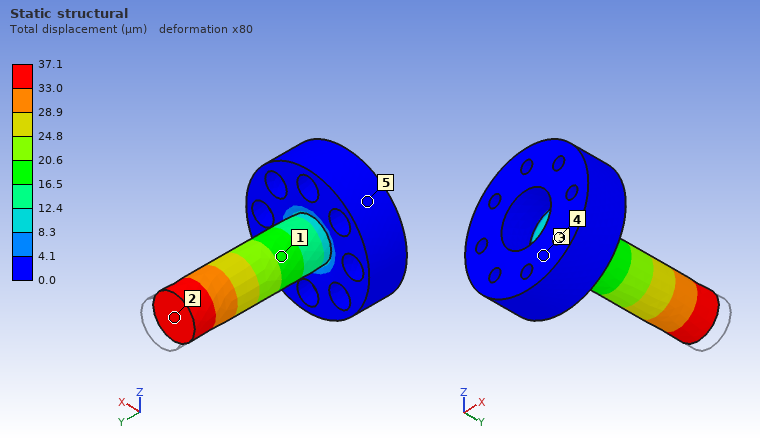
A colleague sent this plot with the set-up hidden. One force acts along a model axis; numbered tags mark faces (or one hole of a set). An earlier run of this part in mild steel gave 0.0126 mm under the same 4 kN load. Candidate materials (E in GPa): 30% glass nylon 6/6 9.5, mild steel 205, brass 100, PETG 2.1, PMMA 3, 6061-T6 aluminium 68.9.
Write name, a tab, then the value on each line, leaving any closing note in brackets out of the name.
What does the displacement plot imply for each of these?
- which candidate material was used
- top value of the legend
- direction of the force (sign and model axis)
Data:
which candidate material was used	6061-T6 aluminium
top value of the legend	37.1 µm
direction of the force	-Y
